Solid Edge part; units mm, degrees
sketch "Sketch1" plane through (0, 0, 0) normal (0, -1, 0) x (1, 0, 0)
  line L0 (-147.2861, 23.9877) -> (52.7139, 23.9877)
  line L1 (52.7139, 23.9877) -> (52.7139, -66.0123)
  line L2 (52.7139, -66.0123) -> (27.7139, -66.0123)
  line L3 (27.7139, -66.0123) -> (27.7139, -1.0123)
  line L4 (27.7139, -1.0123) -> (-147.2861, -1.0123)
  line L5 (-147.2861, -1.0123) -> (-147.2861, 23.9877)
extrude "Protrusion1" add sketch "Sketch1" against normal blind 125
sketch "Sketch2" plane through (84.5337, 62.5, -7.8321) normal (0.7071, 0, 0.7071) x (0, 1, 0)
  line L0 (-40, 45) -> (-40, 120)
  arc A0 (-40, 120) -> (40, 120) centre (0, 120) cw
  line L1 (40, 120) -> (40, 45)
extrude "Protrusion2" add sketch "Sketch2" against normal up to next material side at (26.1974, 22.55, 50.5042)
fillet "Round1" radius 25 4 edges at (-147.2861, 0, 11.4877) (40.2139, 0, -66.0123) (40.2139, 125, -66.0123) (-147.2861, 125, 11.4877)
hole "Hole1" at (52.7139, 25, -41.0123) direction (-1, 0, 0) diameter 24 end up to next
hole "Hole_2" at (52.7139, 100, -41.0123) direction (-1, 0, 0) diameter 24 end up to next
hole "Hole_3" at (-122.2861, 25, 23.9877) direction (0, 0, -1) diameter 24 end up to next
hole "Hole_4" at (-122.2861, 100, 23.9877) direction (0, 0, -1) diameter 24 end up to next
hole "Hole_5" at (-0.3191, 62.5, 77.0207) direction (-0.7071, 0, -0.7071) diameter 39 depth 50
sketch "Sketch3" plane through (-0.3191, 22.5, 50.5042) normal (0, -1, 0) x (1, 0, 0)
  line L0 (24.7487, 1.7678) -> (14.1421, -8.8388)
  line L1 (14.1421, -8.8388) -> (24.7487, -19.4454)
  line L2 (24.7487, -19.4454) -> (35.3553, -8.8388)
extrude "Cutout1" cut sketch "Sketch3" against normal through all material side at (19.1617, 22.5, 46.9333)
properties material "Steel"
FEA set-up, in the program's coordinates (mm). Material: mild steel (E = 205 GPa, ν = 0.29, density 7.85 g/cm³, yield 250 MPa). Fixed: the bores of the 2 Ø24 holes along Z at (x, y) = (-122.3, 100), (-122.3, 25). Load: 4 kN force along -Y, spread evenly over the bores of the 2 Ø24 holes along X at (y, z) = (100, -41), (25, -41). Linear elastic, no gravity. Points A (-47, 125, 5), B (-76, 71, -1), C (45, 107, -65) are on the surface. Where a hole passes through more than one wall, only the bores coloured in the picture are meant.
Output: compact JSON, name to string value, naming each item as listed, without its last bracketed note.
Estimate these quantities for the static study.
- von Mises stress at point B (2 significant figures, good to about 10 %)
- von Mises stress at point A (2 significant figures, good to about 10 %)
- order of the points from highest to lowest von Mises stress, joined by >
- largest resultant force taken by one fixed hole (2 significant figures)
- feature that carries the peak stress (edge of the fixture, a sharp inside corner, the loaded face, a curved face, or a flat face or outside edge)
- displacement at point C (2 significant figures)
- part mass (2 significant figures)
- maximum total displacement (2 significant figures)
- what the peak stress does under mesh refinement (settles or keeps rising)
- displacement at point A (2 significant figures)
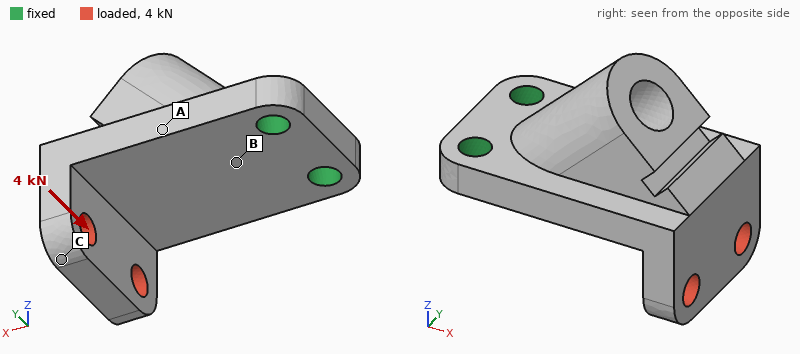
{"von Mises stress at point B": "10 MPa", "von Mises stress at point A": "5.9 MPa", "order of the points from highest to lowest von Mises stress, joined by >": "B > A > C", "largest resultant force taken by one fixed hole": "7.8 kN", "feature that carries the peak stress": "edge of the fixture", "displacement at point C": "29 µm", "part mass": "9.0 kg", "maximum total displacement": "29 µm", "what the peak stress does under mesh refinement": "keeps rising", "displacement at point A": "8.0 µm"}
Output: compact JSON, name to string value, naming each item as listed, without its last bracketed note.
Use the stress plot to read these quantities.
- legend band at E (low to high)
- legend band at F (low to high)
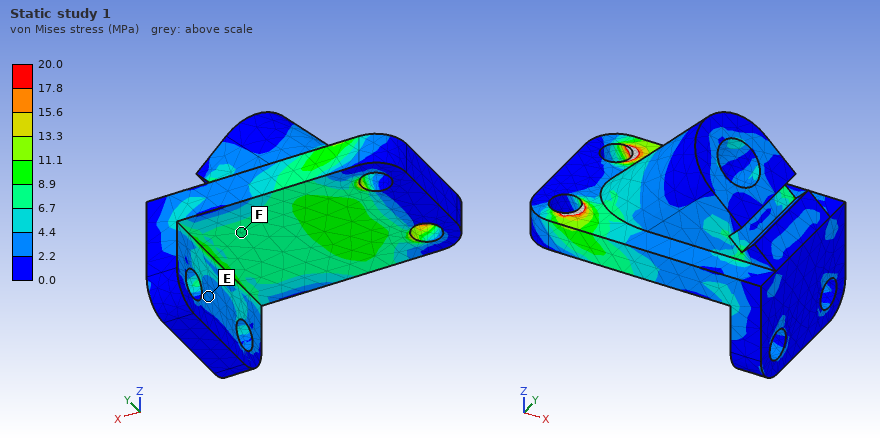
{"legend band at E": "2.2 to 4.4 MPa", "legend band at F": "6.7 to 8.9 MPa"}
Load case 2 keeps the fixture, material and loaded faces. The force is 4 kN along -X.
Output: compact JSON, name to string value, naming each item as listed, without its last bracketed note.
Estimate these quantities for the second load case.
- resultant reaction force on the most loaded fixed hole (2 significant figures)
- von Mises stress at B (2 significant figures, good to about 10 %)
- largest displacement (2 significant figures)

{"resultant reaction force on the most loaded fixed hole": "2.0 kN", "von Mises stress at B": "8.5 MPa", "largest displacement": "59 µm"}
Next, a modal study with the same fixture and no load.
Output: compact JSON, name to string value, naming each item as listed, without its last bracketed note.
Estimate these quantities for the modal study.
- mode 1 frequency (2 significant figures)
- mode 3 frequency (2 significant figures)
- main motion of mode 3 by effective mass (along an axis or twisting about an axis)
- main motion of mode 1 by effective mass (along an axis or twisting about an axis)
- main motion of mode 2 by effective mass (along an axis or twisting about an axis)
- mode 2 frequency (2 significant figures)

{"mode 1 frequency": "530 Hz", "mode 3 frequency": "2000 Hz", "main motion of mode 3 by effective mass": "along Y", "main motion of mode 1 by effective mass": "along Z", "main motion of mode 2 by effective mass": "along Y", "mode 2 frequency": "1500 Hz"}
